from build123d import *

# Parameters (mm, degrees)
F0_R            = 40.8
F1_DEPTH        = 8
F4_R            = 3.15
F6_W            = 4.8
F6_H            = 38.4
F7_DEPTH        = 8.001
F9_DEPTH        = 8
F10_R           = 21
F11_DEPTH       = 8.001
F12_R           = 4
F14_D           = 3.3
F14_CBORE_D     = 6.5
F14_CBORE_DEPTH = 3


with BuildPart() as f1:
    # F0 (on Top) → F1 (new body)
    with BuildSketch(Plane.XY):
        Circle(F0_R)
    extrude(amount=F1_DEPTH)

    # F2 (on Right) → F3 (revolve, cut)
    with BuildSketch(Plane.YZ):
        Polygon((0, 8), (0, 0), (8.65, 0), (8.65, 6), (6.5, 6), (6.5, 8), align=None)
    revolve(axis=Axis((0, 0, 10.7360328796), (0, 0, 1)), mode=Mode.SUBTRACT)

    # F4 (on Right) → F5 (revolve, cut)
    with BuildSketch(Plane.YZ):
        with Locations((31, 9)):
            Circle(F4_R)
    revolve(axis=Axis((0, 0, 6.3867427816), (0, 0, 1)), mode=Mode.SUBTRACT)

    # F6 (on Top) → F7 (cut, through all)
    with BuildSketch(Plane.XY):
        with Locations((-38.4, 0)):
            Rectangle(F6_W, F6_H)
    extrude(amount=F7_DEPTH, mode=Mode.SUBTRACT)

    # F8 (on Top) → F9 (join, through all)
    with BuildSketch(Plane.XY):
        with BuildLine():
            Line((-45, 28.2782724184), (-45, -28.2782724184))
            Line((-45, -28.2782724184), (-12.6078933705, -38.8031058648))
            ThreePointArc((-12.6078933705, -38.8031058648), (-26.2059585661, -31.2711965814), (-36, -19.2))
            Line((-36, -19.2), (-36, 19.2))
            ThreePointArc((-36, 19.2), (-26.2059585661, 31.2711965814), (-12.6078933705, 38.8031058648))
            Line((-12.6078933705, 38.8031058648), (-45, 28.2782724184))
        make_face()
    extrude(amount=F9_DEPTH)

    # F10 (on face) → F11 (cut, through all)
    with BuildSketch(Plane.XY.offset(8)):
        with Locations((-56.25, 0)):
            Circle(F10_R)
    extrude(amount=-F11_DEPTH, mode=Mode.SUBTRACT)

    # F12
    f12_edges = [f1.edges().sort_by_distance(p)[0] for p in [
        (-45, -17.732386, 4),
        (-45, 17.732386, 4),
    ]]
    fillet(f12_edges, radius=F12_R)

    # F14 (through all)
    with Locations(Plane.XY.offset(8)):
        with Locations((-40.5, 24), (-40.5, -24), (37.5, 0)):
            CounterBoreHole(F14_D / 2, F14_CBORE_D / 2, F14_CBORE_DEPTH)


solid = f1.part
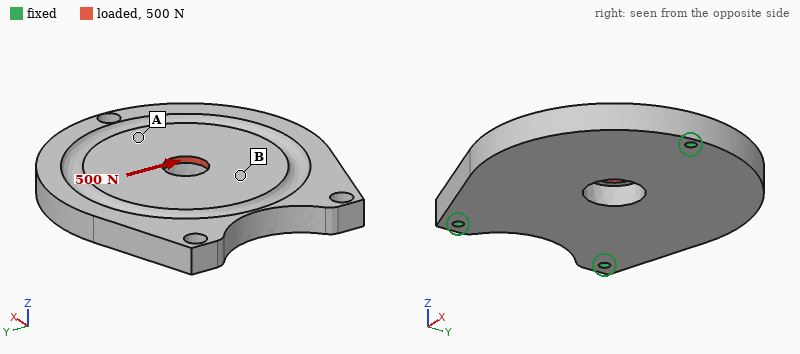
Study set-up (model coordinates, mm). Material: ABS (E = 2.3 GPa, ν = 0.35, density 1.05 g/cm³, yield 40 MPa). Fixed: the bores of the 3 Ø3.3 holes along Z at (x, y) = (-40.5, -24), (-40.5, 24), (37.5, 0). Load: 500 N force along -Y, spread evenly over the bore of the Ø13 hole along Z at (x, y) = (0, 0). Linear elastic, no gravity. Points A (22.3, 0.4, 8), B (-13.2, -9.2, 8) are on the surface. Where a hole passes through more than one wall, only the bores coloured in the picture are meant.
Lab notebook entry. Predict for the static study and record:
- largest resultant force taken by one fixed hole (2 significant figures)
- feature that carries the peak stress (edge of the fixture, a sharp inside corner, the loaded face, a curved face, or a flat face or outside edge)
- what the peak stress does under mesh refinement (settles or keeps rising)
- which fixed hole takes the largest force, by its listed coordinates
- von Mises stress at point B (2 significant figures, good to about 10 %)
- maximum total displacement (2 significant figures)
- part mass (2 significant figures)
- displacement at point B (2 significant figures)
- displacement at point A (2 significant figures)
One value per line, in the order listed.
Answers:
220 N
edge of the fixture
keeps rising
(37.5, 0)
2.7 MPa
0.17 mm
43 g
0.053 mm
0.047 mm
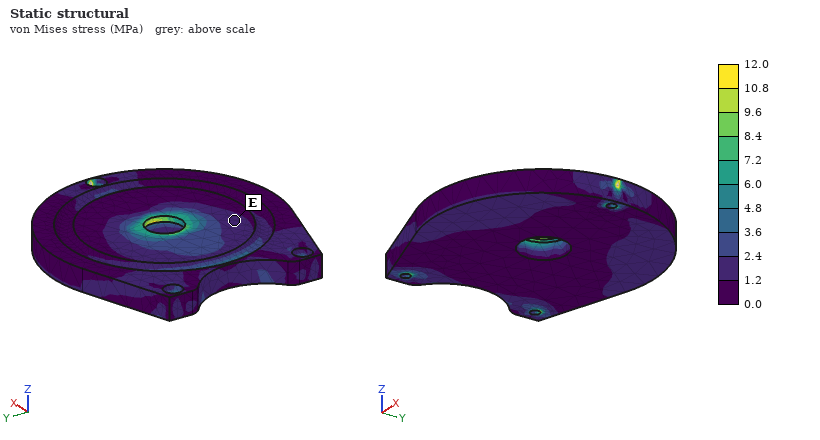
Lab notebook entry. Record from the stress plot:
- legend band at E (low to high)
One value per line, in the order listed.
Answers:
1.2 to 2.4 MPa
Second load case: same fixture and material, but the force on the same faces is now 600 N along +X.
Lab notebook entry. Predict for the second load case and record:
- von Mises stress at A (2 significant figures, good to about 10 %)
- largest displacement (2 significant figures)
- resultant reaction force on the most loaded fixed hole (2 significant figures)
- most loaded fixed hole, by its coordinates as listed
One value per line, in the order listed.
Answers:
2.2 MPa
55 µm
240 N
(37.5, 0)
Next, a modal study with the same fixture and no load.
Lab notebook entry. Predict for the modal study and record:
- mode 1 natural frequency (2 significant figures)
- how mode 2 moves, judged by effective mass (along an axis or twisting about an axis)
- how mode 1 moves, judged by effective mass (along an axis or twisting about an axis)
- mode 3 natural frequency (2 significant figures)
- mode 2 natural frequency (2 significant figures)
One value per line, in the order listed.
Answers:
870 Hz
along Z
twisting about X
2200 Hz
980 Hz
